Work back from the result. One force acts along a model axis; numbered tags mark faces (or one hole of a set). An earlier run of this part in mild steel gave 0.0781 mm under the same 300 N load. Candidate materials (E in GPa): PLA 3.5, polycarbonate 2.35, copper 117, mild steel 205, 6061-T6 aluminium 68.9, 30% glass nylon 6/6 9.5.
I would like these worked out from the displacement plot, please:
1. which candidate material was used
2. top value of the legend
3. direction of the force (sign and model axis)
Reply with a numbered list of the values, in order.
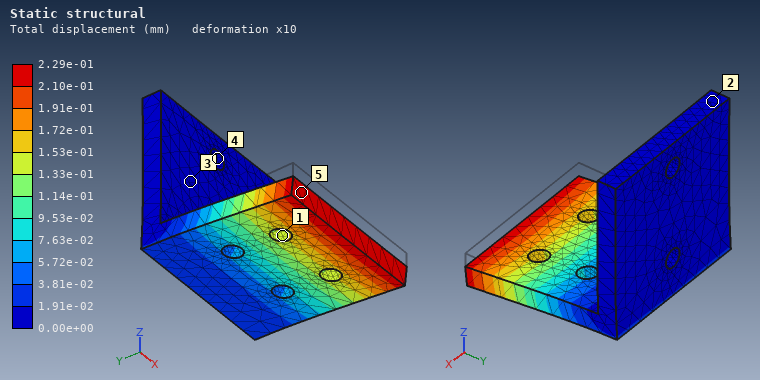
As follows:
1. 6061-T6 aluminium
2. 2.29e-01 mm
3. -Z
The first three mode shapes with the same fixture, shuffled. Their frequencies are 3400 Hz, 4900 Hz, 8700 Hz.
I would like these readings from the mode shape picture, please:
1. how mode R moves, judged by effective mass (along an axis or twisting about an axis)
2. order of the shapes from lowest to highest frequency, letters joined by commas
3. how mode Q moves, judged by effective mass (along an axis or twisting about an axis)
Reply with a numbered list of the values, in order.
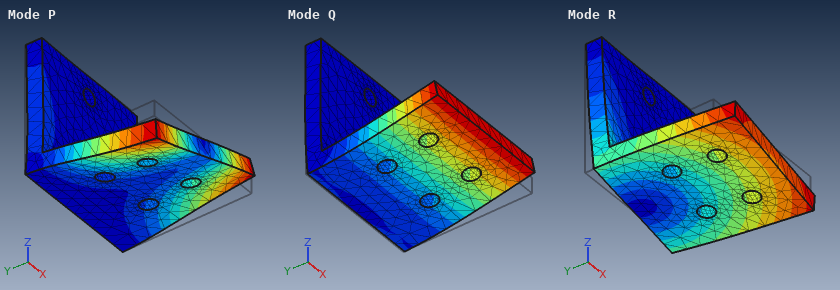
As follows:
1. along X
2. Q, R, P
3. along Z
